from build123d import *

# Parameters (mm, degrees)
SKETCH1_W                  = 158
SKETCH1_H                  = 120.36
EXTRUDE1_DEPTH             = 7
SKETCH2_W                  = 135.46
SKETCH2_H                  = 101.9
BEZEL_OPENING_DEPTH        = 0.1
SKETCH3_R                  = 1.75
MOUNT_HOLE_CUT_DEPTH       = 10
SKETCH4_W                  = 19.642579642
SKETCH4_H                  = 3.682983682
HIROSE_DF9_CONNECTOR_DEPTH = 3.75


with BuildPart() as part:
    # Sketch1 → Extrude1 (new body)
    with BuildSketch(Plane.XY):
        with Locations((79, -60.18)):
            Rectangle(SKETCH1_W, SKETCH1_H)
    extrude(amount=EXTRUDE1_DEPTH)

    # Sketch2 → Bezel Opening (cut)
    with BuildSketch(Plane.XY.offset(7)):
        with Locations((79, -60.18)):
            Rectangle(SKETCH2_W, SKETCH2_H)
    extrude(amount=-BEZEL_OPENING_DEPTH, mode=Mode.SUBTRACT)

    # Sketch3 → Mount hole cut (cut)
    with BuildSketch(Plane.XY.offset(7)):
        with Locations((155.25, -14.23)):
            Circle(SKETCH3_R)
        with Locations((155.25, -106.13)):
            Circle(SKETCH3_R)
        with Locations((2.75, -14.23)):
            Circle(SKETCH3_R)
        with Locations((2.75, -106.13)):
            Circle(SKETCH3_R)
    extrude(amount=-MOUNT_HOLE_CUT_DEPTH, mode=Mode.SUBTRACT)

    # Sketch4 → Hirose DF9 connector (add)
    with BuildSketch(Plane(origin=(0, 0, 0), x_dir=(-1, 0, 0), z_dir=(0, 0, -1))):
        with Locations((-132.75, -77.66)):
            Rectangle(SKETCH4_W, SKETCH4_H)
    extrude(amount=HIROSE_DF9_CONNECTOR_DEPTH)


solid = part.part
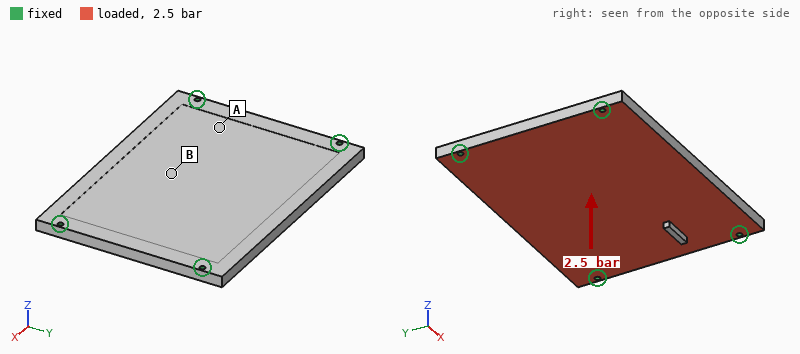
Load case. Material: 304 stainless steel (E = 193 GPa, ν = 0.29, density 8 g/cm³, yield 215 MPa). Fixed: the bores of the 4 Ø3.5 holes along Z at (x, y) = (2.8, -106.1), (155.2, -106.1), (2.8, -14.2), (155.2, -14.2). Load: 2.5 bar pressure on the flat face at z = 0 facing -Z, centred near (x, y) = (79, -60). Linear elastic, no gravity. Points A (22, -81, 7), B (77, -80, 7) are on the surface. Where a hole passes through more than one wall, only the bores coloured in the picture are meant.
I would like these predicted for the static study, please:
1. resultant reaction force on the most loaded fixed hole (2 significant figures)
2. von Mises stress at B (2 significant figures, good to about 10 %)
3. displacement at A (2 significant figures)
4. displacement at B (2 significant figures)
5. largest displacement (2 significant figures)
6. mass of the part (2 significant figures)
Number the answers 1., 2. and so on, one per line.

1. 1.2 kN
2. 37 MPa
3. 0.048 mm
4. 0.12 mm
5. 0.13 mm
6. 1.1 kg
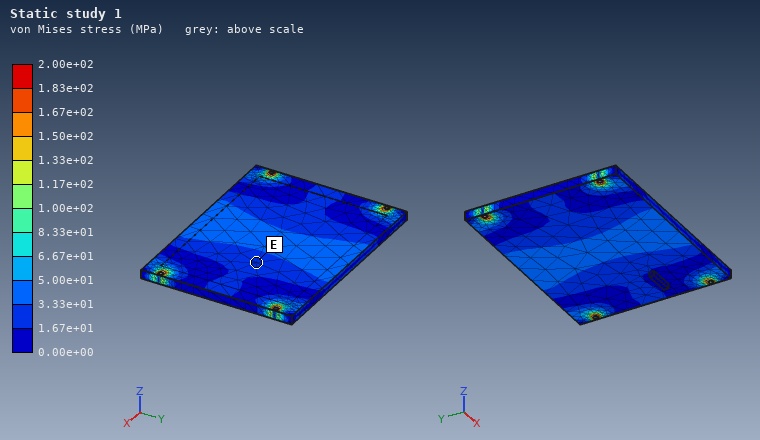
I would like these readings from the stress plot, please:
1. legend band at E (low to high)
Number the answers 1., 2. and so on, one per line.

1. 1.67e+01 to 3.33e+01 MPa
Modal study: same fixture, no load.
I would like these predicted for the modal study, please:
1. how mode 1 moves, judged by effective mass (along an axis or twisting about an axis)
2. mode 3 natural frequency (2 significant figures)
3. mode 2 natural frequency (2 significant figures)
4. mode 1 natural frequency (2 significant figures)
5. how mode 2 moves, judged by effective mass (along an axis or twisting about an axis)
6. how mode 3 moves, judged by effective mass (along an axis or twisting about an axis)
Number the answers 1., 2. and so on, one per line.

1. along Z
2. 2900 Hz
3. 1700 Hz
4. 1100 Hz
5. twisting about X
6. twisting about Y
